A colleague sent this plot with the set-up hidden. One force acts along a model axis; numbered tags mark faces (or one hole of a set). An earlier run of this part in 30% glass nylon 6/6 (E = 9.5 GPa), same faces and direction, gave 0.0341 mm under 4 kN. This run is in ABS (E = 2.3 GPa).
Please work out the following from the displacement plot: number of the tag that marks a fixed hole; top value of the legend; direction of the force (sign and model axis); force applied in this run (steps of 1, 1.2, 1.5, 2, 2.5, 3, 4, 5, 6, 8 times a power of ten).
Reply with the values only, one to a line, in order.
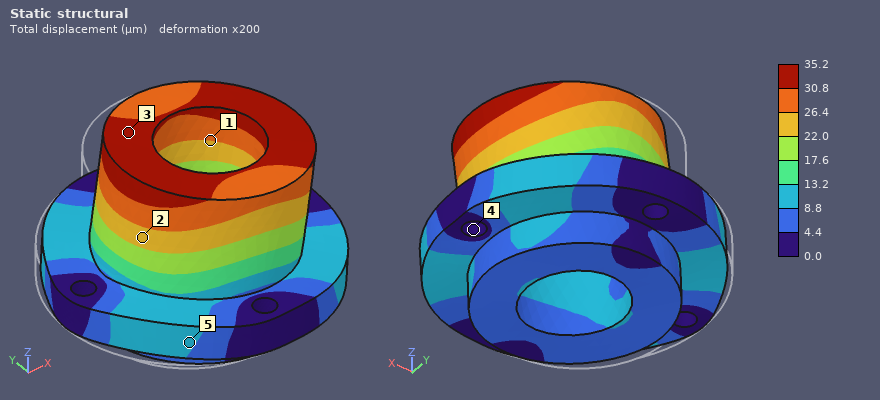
4
35.2 µm
+X
1 kN
